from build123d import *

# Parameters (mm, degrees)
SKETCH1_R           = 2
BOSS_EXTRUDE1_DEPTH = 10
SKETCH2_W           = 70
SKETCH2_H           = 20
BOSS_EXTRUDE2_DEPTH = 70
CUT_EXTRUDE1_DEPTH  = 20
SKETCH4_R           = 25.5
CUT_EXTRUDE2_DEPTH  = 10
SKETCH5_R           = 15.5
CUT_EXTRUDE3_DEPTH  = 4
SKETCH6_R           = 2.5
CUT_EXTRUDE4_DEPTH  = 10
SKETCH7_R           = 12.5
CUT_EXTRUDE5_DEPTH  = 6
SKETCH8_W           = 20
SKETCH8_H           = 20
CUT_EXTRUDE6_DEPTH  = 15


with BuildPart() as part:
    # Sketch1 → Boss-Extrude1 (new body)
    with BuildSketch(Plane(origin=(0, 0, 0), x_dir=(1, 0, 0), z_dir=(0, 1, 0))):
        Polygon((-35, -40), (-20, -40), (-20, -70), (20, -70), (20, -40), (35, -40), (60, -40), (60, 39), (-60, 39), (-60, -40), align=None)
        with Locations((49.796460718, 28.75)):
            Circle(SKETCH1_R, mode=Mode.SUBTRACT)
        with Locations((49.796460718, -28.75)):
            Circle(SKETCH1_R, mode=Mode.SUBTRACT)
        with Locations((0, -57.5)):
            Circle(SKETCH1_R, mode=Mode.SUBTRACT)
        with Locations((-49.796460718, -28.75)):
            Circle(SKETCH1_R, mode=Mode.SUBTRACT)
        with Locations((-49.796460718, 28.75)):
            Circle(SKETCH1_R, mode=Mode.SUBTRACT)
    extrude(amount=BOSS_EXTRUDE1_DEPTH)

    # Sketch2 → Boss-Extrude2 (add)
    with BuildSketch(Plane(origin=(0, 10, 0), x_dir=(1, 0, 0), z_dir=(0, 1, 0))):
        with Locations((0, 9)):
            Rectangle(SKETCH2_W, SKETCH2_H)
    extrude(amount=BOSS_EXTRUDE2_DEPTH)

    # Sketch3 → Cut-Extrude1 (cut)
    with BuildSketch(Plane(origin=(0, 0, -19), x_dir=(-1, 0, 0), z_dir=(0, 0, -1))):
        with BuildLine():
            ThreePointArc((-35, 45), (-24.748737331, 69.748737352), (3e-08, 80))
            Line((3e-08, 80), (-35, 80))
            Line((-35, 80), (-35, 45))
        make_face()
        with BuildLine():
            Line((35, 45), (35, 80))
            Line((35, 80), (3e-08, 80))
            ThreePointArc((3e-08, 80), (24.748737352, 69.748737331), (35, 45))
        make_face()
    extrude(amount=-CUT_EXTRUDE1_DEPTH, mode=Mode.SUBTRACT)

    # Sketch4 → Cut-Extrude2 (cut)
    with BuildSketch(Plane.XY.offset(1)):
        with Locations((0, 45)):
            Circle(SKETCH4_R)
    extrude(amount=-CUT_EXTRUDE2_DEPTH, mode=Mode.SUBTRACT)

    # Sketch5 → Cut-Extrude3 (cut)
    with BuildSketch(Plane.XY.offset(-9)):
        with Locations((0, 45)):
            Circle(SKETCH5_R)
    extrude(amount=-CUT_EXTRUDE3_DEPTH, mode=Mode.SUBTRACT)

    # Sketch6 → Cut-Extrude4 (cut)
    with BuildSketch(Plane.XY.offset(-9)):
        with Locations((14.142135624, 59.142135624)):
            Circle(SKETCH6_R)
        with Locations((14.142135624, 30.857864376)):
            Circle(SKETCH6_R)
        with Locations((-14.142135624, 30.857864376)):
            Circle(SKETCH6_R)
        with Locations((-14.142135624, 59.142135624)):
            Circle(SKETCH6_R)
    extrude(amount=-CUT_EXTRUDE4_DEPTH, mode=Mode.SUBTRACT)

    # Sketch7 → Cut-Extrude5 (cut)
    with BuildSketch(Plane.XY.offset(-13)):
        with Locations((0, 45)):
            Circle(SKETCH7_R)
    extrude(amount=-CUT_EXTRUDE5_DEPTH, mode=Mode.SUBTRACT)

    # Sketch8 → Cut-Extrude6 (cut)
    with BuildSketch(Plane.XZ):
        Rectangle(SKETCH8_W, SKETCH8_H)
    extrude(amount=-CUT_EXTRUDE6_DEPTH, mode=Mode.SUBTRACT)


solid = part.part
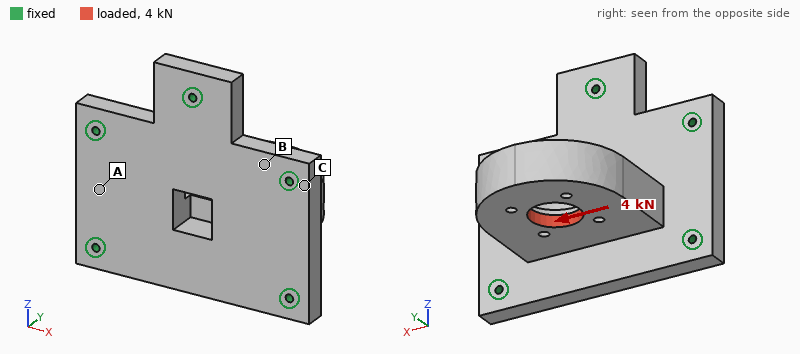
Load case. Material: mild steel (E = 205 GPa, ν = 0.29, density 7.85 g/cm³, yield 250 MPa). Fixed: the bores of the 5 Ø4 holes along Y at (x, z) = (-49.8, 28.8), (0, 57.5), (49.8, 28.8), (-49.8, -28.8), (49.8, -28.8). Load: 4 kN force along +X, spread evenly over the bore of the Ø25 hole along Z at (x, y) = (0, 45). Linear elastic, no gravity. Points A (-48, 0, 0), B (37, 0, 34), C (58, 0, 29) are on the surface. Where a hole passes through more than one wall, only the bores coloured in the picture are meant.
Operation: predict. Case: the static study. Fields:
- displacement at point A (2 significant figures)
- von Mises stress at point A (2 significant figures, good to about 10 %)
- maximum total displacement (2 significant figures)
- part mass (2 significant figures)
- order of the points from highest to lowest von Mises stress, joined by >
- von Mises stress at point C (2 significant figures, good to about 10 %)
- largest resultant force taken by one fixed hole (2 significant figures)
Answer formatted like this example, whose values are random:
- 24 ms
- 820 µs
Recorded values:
- 3.5 µm
- 12 MPa
- 18 µm
- 1.3 kg
- A > C > B
- 6.9 MPa
- 1.8 kN
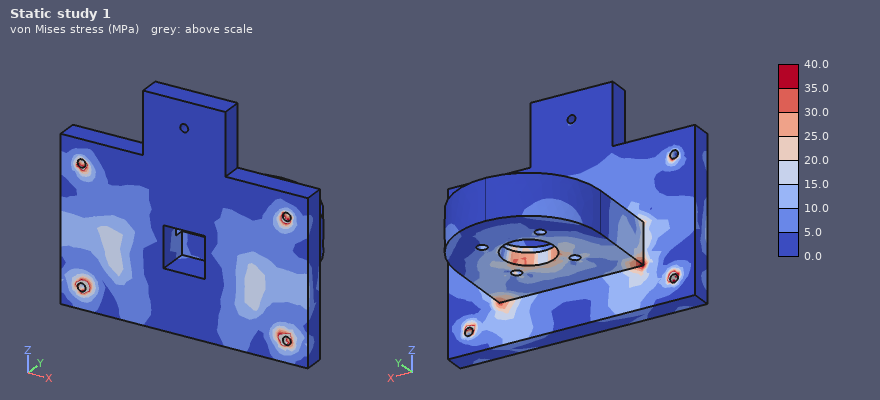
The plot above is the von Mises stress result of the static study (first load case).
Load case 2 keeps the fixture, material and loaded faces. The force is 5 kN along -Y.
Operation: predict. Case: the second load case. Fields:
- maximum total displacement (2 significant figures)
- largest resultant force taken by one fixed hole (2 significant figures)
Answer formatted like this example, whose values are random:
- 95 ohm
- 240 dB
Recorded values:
- 24 µm
- 2.1 kN
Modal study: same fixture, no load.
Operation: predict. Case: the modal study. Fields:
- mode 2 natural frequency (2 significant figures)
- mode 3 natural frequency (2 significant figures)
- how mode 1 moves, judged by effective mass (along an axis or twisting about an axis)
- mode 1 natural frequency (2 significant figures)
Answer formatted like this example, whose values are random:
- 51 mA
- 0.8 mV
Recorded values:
- 4000 Hz
- 4100 Hz
- along Z
- 2100 Hz
